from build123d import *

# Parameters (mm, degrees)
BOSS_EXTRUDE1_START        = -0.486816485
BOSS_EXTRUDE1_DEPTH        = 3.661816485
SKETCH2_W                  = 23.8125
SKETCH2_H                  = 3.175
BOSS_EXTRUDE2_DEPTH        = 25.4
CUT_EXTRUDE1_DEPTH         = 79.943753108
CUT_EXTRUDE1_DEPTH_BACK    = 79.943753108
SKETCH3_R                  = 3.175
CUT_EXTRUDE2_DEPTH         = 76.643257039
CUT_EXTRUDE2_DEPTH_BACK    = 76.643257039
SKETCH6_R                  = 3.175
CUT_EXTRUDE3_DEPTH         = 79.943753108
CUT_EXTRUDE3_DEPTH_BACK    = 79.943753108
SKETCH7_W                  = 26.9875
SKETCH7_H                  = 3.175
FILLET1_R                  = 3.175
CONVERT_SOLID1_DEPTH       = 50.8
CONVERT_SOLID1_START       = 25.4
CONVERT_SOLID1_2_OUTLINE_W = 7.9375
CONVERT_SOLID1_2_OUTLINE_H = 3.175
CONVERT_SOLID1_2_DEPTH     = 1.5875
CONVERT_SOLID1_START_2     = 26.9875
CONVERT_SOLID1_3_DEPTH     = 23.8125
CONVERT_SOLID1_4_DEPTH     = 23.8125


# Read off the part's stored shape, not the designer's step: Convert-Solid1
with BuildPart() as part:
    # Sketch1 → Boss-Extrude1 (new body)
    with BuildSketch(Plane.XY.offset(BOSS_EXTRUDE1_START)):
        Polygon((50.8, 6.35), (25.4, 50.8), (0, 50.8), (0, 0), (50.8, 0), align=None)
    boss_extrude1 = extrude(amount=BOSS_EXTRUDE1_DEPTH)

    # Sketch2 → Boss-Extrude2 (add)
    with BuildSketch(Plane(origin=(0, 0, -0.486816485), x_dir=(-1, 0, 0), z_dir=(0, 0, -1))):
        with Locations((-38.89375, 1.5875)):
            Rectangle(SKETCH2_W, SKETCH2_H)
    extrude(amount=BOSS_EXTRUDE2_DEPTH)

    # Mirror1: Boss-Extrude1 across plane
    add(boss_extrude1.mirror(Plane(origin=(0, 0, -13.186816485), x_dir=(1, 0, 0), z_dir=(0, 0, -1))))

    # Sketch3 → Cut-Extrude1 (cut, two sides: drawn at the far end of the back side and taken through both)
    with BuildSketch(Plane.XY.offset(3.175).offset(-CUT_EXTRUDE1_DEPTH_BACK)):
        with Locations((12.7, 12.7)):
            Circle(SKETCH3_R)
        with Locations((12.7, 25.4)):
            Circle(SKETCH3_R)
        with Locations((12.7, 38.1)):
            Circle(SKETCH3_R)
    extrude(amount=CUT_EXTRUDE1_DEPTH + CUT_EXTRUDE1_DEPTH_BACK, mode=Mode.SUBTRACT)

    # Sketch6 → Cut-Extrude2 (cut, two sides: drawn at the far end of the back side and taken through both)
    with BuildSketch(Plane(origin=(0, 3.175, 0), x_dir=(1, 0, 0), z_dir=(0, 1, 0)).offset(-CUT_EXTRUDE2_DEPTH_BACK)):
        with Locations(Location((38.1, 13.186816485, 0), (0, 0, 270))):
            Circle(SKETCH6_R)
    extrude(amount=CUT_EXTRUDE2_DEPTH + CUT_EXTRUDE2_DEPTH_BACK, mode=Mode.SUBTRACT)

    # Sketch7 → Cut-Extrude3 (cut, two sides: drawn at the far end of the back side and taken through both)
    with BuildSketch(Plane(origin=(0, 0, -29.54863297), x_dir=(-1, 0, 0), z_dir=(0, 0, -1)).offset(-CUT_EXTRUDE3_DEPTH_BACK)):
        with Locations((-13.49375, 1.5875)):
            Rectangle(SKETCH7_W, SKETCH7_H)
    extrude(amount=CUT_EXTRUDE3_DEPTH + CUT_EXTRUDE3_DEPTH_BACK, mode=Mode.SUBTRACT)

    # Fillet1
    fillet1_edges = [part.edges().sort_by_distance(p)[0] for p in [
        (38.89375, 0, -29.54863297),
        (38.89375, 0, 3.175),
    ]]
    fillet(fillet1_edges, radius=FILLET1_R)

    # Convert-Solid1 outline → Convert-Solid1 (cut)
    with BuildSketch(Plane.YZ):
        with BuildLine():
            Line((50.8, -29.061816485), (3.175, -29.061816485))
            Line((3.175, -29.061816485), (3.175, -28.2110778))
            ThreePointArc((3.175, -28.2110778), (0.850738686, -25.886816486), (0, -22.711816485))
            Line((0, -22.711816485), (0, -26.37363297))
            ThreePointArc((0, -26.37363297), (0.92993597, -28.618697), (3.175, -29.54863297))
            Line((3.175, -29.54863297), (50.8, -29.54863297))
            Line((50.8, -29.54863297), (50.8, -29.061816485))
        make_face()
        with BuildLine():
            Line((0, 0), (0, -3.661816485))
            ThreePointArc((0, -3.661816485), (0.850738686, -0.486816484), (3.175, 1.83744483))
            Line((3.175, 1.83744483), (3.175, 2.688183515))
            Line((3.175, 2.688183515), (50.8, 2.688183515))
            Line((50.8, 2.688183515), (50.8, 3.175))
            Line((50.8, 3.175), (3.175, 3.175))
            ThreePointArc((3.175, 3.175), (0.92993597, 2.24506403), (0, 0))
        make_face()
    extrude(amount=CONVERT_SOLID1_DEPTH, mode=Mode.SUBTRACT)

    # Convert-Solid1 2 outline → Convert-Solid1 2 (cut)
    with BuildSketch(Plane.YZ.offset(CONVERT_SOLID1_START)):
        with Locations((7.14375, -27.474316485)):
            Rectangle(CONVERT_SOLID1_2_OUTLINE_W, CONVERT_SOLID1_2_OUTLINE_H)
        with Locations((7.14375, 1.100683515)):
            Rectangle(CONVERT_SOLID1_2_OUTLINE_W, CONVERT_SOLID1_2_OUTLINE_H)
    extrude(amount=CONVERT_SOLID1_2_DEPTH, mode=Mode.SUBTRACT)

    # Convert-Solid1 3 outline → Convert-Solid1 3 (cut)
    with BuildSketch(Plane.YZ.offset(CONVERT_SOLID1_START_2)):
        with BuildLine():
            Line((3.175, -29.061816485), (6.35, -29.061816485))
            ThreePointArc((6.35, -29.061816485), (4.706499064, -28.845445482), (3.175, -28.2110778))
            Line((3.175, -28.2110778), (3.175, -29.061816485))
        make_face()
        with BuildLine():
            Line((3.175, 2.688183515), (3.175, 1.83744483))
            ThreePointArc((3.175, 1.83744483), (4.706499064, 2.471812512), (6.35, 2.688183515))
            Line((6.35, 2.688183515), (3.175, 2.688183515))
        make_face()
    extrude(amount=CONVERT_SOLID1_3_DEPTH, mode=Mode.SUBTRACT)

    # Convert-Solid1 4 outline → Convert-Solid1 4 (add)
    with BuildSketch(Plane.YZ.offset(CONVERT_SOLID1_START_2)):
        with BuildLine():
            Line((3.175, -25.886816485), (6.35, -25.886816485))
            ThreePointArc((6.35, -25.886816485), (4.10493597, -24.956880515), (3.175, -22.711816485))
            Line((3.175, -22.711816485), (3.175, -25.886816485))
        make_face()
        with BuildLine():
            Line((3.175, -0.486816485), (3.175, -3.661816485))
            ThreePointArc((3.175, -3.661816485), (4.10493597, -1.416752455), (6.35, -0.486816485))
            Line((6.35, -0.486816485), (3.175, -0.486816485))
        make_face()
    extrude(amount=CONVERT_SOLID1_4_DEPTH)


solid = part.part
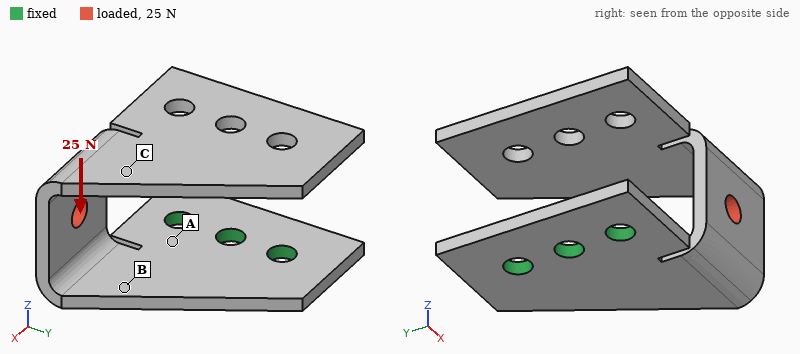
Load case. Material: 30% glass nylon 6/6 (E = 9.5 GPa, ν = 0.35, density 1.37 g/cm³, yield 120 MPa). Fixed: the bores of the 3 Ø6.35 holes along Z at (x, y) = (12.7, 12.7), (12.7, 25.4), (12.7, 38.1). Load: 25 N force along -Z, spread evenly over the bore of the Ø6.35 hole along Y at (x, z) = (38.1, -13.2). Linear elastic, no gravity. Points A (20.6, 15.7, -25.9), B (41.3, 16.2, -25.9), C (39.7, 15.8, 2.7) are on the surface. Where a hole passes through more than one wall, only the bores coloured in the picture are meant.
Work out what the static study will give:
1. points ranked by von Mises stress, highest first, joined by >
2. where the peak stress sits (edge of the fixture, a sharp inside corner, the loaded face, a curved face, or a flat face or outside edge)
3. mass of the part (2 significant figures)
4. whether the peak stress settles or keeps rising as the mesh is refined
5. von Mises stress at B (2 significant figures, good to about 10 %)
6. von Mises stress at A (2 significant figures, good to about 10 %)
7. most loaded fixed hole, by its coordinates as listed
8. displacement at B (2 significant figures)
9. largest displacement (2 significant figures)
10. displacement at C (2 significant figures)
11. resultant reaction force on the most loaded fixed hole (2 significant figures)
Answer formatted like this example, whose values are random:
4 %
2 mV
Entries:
A > B > C
a sharp inside corner
18 g
keeps rising
7.0 MPa
11 MPa
(12.7, 12.7)
0.19 mm
0.90 mm
0.54 mm
33 N
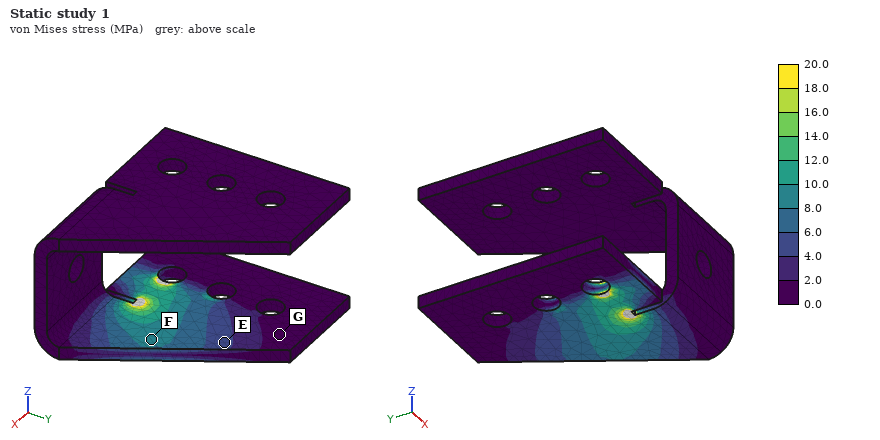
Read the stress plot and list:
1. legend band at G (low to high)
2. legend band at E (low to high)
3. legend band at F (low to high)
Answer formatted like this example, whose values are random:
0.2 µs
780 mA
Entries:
0.0 to 2.0 MPa
4.0 to 6.0 MPa
8.0 to 10.0 MPa
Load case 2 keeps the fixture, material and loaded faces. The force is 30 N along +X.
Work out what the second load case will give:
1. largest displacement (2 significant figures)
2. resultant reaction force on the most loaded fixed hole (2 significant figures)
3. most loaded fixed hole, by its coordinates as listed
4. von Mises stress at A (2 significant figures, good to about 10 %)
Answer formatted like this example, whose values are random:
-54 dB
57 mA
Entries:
0.89 mm
36 N
(12.7, 12.7)
9.3 MPa
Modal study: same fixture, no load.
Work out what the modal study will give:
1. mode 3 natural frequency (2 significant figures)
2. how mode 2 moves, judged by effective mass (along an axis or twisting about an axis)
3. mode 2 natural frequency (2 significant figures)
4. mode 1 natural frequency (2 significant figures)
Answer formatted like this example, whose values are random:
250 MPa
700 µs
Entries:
400 Hz
along X
210 Hz
170 Hz
